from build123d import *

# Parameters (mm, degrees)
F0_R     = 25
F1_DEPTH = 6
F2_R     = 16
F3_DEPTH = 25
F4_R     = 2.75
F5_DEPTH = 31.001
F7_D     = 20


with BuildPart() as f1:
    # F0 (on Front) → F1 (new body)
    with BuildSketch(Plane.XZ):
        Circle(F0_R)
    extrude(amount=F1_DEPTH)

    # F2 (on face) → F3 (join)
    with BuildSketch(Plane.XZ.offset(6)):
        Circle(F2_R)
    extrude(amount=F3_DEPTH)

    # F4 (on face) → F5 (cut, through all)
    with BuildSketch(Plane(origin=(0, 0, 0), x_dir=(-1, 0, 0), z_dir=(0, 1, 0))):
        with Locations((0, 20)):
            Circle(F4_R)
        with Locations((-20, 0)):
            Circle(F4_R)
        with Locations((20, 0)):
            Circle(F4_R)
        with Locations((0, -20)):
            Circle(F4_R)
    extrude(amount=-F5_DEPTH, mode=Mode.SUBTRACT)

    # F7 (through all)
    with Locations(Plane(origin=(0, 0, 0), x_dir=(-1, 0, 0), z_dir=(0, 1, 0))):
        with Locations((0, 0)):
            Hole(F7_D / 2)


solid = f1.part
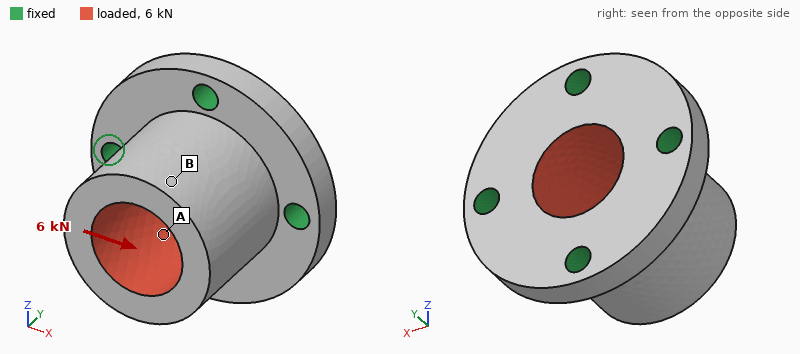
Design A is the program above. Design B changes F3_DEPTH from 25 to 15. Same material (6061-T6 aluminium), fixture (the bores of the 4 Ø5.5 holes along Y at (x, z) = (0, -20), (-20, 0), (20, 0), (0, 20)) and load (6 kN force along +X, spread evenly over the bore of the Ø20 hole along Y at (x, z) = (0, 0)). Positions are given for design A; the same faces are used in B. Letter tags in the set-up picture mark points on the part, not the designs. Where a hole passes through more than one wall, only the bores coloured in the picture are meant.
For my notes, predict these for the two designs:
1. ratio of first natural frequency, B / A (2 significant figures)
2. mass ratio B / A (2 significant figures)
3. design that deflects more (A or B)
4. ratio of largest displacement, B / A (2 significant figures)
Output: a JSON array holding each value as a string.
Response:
["1.7", "0.77", "A", "0.50"]
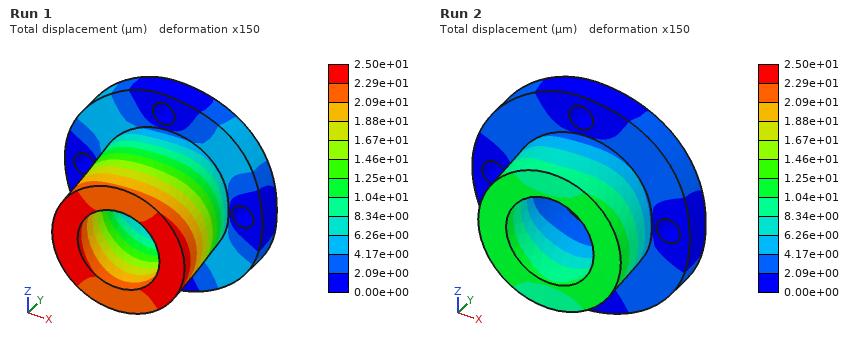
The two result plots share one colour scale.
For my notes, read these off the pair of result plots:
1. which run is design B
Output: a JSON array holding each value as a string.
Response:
["Run 2"]
